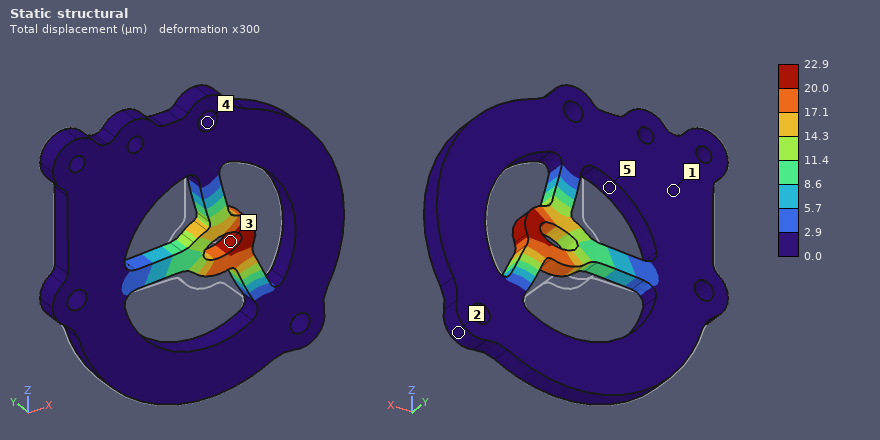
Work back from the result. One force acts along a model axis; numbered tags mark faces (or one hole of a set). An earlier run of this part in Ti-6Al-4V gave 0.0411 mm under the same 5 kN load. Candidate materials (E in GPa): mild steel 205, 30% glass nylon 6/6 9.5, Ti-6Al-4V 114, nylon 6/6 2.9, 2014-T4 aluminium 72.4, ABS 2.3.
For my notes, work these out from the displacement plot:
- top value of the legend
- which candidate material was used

22.9 µm
mild steel
